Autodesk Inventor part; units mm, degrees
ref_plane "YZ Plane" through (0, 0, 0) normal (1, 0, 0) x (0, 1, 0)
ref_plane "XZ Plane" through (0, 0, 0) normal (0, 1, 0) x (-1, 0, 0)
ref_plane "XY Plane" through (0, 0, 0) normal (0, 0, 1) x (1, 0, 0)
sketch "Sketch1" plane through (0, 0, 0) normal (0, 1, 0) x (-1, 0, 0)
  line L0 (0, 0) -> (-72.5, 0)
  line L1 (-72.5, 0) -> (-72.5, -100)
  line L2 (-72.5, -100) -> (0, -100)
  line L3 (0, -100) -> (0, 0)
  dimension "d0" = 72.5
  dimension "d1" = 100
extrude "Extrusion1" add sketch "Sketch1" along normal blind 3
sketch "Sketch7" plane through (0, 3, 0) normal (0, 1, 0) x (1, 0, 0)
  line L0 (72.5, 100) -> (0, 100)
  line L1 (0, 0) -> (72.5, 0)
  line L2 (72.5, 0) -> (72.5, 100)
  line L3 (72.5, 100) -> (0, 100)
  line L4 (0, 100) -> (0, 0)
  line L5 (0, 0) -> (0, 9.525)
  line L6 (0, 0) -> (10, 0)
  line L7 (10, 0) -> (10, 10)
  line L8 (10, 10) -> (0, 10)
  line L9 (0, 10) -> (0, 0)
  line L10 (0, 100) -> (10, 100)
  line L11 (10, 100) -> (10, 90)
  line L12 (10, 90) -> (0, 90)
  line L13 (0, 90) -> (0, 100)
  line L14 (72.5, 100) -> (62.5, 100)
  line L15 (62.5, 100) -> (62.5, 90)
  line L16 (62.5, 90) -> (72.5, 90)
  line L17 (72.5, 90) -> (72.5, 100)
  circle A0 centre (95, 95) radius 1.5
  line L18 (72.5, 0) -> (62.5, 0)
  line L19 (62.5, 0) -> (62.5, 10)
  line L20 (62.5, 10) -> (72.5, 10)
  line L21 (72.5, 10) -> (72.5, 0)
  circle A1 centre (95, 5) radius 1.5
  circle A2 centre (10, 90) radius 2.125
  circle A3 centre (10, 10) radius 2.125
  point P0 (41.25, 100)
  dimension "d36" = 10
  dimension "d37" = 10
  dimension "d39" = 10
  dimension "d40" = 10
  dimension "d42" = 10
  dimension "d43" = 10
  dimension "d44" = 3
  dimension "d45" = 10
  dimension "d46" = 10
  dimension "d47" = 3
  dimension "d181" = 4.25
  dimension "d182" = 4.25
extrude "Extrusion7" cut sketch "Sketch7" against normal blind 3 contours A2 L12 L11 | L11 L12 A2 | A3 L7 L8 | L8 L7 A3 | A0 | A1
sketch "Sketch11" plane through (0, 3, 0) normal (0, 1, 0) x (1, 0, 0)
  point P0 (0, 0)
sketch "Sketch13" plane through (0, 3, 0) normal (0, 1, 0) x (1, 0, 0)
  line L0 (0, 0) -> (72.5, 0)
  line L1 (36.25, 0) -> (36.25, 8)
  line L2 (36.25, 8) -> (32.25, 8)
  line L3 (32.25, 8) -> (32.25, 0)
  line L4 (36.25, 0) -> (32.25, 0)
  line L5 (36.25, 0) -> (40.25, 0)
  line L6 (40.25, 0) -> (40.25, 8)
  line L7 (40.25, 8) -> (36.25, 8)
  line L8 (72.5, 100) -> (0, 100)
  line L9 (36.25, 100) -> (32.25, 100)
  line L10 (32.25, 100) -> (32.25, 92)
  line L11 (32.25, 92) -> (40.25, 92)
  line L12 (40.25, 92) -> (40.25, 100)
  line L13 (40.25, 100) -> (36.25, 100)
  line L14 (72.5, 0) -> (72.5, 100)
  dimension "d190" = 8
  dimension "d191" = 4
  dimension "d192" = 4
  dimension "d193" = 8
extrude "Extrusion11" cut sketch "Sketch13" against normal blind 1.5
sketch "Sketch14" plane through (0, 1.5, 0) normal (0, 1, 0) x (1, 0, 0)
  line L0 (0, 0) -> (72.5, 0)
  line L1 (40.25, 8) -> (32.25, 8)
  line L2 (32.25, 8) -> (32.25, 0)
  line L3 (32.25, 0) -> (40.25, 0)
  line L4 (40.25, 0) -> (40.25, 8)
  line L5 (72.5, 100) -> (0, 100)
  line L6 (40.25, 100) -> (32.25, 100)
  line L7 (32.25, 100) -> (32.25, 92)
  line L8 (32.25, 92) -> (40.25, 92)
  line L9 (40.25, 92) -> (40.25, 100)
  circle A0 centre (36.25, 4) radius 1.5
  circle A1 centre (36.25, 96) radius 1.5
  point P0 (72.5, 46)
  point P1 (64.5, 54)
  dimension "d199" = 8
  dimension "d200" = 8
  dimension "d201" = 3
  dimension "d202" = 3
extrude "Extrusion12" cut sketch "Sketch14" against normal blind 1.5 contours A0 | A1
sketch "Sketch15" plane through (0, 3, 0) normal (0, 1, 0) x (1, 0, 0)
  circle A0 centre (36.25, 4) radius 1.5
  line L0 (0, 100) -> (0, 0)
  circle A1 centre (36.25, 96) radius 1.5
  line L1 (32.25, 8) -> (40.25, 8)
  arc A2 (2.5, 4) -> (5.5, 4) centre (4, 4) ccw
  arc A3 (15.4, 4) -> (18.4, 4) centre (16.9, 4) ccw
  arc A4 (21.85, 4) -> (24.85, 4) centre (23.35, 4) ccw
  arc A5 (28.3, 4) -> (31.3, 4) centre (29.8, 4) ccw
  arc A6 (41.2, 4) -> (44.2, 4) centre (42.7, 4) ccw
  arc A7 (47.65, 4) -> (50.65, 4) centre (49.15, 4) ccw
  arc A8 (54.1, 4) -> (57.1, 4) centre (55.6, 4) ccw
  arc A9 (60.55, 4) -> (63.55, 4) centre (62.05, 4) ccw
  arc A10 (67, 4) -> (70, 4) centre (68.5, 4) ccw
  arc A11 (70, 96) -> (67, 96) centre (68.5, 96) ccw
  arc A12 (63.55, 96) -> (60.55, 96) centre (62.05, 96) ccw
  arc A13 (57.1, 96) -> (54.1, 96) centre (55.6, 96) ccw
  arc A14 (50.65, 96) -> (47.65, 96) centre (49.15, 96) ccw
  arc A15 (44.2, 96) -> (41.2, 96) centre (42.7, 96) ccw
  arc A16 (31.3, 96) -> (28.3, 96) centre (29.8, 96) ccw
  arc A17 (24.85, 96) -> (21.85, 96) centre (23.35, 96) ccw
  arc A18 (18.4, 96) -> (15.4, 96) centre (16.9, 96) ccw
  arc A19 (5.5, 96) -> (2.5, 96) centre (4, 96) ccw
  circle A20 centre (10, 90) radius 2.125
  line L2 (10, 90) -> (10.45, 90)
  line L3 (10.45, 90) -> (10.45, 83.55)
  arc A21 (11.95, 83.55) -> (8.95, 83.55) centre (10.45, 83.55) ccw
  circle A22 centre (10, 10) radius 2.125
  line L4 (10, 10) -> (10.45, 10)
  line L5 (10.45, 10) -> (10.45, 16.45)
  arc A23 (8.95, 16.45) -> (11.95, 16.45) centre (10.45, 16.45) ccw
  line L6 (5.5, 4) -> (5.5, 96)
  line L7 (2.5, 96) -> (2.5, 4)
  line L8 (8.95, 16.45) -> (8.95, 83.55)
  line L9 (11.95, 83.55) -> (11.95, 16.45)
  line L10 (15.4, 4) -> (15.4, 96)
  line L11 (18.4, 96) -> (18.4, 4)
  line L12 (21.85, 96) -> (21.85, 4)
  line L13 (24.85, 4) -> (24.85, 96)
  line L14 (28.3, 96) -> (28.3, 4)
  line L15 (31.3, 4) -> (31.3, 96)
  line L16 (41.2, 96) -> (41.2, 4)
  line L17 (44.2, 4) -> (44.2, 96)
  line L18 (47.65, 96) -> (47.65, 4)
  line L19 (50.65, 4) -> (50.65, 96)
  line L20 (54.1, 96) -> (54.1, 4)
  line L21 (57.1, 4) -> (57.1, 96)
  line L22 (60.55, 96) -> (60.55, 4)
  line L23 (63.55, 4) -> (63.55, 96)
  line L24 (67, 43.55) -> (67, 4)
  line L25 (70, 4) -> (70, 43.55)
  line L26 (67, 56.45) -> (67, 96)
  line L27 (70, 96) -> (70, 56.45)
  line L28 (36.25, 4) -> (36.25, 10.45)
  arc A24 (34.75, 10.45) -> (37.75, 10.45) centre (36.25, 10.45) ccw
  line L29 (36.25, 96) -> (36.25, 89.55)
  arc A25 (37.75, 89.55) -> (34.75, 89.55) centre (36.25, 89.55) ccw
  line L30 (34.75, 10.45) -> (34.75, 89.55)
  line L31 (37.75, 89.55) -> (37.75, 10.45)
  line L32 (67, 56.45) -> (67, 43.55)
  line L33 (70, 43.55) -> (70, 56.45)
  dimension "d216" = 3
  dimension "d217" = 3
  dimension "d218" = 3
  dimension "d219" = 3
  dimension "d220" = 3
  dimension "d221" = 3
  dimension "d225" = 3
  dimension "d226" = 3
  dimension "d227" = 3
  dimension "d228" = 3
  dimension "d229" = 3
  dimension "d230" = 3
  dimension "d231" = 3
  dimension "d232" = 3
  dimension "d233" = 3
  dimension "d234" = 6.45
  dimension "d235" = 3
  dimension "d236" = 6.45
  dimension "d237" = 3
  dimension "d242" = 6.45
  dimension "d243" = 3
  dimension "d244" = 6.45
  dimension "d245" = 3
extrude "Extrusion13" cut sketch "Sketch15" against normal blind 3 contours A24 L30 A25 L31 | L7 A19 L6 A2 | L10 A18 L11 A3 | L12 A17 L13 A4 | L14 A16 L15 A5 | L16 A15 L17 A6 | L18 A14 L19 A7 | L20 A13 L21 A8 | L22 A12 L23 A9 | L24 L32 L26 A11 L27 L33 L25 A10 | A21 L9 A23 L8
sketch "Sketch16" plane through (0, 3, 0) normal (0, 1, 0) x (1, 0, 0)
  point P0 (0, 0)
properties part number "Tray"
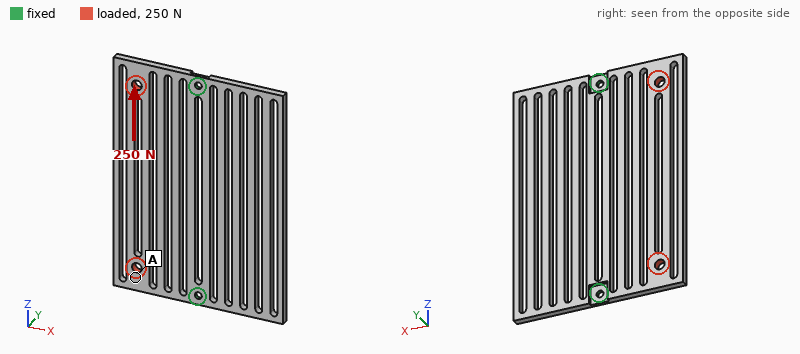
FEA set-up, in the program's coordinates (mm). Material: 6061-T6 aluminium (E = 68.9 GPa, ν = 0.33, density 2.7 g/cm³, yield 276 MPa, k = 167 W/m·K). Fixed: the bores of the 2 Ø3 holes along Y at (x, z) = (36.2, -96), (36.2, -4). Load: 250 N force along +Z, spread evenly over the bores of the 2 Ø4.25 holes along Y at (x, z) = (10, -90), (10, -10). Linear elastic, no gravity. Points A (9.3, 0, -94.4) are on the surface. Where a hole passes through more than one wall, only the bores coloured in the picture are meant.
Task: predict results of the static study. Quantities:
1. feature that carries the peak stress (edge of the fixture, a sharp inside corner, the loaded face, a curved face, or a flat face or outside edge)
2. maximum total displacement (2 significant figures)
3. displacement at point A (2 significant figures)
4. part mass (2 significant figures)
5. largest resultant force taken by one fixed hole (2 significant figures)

a curved face
0.25 mm
0.20 mm
34 g
130 N
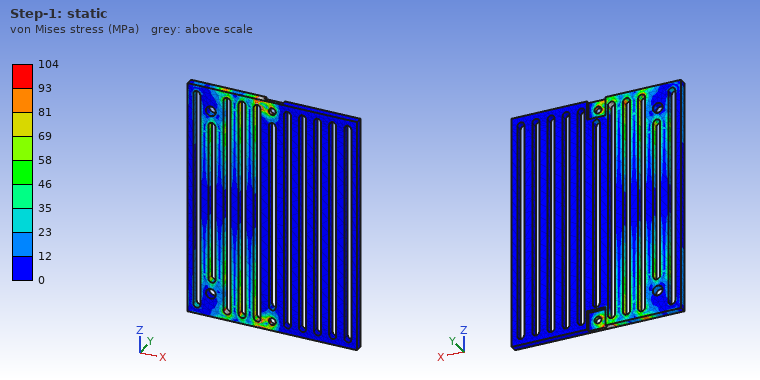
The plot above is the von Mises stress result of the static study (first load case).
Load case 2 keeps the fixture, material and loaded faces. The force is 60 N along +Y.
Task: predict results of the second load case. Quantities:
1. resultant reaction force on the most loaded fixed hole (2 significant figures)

36 N
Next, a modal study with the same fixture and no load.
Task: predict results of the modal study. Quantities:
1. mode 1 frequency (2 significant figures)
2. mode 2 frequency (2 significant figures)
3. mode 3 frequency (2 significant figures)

390 Hz
400 Hz
1100 Hz
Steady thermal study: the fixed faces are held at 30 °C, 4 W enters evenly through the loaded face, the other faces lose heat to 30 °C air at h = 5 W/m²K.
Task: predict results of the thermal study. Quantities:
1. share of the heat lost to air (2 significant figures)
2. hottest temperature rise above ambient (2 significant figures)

18 %
29 K
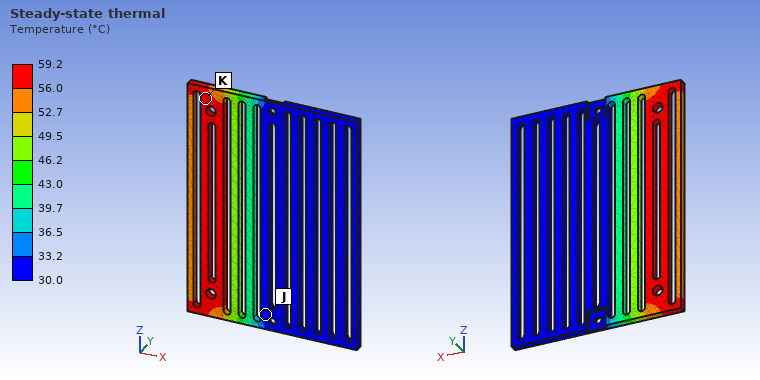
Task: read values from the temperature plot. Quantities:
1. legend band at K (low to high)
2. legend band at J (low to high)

56.0 to 59.2 °C
30.0 to 33.2 °C
